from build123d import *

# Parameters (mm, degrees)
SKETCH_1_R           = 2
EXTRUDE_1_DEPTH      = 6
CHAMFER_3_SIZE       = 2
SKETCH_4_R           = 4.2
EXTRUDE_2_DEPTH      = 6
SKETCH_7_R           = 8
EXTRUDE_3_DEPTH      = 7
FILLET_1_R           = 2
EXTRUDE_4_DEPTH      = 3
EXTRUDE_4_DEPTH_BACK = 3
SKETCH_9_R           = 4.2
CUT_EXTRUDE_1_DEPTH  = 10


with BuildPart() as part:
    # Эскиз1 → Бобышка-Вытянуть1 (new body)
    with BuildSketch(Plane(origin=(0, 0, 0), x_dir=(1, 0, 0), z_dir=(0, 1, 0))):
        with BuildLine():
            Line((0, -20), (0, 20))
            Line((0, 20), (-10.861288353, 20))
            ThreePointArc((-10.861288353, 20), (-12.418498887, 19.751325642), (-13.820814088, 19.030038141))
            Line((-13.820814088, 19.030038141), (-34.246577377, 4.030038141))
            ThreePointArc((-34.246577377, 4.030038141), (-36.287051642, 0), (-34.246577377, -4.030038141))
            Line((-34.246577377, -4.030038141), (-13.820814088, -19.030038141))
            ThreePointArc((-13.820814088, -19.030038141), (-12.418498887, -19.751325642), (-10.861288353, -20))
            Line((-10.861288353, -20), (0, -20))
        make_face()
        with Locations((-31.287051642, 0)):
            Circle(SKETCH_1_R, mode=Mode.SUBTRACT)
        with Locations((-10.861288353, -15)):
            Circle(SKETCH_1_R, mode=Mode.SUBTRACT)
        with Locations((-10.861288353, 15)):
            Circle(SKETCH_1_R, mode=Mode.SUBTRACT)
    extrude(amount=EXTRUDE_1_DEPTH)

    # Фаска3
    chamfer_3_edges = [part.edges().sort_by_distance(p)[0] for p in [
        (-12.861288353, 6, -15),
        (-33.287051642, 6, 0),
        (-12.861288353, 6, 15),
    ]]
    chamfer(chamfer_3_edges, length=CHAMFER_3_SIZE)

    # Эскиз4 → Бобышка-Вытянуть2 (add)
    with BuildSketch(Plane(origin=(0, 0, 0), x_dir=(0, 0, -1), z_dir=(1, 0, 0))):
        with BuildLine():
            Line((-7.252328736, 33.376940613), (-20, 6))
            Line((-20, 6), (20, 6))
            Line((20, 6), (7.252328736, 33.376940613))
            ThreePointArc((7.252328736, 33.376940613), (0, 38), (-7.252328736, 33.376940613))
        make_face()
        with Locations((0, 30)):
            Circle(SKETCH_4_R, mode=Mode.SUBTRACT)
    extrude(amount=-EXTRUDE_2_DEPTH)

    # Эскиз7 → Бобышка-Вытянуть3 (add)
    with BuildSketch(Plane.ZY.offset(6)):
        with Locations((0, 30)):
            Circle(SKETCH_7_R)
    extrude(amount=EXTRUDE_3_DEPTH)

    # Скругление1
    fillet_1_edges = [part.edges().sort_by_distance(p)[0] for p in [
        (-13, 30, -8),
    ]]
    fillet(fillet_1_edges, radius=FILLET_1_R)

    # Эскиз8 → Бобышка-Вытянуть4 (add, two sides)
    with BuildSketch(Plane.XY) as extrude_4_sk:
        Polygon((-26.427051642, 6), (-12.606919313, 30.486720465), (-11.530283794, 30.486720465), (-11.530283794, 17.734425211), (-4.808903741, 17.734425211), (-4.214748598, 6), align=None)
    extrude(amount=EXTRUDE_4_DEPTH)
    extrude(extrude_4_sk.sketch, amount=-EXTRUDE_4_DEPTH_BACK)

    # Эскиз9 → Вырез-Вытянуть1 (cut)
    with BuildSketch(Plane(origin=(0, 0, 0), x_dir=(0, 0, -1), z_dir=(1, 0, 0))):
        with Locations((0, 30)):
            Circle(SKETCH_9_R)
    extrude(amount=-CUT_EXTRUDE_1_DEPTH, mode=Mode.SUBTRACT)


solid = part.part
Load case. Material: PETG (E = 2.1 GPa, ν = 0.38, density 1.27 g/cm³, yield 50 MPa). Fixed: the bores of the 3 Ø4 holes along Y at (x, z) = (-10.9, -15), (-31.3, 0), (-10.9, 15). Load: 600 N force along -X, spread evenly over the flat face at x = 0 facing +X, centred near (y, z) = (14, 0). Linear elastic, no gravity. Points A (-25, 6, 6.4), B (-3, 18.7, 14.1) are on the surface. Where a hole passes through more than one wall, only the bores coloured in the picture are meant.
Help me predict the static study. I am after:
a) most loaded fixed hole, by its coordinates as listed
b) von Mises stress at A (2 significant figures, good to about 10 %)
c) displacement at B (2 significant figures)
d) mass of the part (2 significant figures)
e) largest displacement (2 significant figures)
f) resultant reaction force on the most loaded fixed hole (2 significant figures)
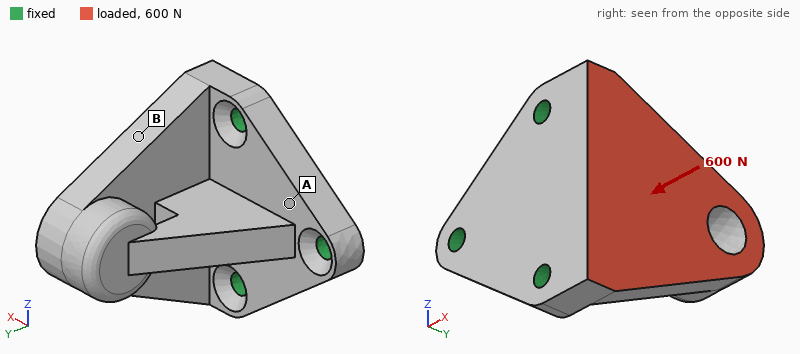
(-31.3, 0)
5.3 MPa
0.26 mm
16 g
0.43 mm
420 N
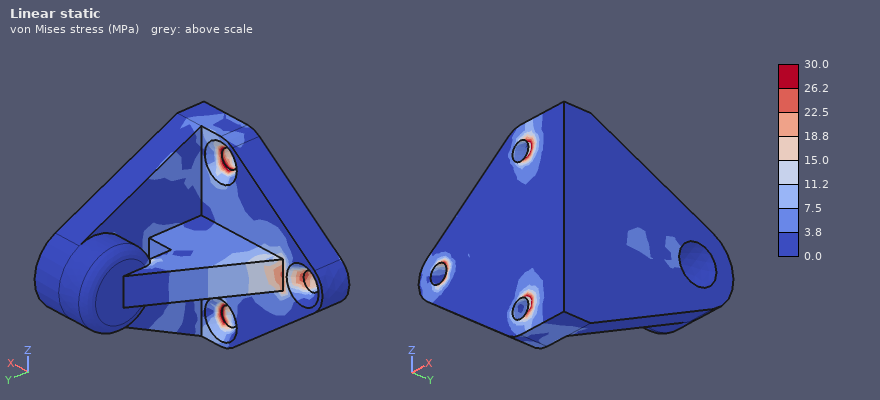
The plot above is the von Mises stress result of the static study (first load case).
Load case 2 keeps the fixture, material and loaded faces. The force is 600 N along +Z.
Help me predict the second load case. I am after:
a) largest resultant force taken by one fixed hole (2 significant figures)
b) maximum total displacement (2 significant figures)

430 N
0.23 mm
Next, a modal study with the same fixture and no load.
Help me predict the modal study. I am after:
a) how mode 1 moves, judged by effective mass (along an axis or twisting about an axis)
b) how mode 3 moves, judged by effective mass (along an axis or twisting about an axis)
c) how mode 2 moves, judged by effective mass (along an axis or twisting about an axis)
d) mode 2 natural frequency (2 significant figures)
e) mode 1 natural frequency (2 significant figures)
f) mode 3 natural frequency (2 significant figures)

along X
along Y
along Z
2500 Hz
2000 Hz
4500 Hz
